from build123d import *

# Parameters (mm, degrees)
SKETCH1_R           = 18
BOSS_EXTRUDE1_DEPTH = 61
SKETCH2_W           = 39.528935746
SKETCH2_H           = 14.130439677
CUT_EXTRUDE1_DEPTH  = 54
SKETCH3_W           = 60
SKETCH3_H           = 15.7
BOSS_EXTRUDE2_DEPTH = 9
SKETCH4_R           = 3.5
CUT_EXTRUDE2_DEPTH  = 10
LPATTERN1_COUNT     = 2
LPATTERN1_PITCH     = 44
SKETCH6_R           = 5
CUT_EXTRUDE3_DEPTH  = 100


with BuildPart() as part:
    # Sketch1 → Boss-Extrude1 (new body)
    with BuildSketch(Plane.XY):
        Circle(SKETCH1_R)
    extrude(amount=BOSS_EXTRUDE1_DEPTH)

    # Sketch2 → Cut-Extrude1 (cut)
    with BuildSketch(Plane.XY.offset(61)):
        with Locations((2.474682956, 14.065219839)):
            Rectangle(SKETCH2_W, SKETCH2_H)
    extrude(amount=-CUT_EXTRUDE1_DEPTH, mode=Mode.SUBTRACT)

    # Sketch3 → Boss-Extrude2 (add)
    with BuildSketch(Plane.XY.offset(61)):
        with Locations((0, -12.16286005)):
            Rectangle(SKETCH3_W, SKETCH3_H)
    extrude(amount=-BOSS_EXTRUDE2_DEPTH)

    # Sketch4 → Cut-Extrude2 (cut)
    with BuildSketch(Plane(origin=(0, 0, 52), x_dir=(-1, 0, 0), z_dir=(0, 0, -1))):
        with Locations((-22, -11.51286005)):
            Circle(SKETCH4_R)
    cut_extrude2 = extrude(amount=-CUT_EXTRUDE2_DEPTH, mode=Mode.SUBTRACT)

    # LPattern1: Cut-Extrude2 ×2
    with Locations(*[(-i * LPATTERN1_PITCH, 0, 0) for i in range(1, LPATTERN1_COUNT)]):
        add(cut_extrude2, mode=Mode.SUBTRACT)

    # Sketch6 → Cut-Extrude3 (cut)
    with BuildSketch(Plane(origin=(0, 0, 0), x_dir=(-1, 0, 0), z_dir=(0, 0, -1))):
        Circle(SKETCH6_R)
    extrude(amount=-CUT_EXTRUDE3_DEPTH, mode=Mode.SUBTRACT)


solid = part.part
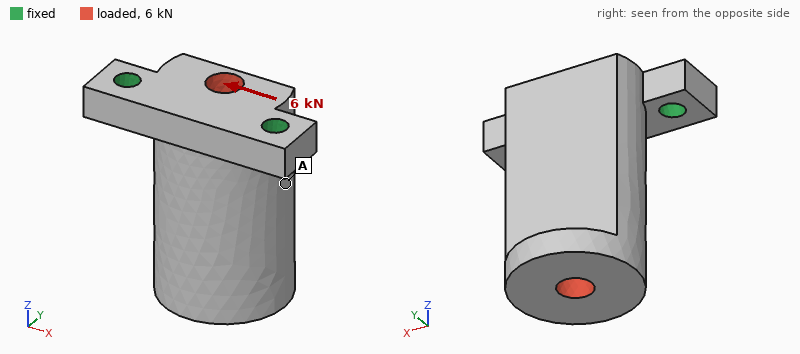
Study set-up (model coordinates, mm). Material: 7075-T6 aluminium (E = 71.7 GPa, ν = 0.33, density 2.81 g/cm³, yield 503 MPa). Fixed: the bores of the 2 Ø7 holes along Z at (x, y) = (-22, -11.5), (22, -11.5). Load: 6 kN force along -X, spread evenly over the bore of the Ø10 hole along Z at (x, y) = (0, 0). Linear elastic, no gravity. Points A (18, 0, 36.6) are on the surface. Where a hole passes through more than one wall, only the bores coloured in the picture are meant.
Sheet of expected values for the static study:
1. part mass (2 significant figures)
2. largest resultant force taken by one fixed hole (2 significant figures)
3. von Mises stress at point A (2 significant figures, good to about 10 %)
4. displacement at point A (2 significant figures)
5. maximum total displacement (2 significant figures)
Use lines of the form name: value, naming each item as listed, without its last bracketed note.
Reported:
part mass: 130 g
largest resultant force taken by one fixed hole: 5.5 kN
von Mises stress at point A: 18 MPa
displacement at point A: 38 µm
maximum total displacement: 94 µm
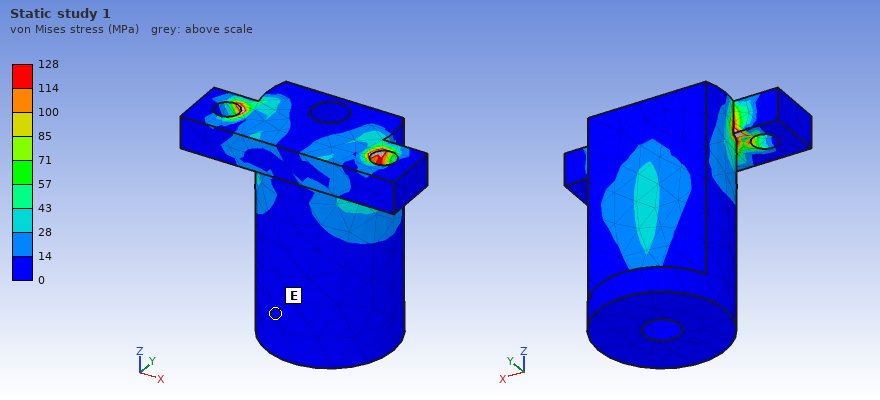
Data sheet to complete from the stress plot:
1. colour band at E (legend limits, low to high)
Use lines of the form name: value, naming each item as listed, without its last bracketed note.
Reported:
colour band at E: 0 to 14 MPa
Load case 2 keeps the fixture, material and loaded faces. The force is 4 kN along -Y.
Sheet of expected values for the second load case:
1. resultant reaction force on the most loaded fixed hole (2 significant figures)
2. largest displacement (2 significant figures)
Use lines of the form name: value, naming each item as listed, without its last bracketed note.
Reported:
resultant reaction force on the most loaded fixed hole: 2.1 kN
largest displacement: 0.41 mm
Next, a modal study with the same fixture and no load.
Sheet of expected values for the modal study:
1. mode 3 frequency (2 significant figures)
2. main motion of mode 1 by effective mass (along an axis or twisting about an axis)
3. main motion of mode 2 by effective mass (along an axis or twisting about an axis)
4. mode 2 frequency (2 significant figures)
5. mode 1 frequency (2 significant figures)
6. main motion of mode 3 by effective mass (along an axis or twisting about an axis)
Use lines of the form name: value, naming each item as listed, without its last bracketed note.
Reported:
mode 3 frequency: 9600 Hz
main motion of mode 1 by effective mass: along Y
main motion of mode 2 by effective mass: along X
mode 2 frequency: 4300 Hz
mode 1 frequency: 1700 Hz
main motion of mode 3 by effective mass: twisting about Z
